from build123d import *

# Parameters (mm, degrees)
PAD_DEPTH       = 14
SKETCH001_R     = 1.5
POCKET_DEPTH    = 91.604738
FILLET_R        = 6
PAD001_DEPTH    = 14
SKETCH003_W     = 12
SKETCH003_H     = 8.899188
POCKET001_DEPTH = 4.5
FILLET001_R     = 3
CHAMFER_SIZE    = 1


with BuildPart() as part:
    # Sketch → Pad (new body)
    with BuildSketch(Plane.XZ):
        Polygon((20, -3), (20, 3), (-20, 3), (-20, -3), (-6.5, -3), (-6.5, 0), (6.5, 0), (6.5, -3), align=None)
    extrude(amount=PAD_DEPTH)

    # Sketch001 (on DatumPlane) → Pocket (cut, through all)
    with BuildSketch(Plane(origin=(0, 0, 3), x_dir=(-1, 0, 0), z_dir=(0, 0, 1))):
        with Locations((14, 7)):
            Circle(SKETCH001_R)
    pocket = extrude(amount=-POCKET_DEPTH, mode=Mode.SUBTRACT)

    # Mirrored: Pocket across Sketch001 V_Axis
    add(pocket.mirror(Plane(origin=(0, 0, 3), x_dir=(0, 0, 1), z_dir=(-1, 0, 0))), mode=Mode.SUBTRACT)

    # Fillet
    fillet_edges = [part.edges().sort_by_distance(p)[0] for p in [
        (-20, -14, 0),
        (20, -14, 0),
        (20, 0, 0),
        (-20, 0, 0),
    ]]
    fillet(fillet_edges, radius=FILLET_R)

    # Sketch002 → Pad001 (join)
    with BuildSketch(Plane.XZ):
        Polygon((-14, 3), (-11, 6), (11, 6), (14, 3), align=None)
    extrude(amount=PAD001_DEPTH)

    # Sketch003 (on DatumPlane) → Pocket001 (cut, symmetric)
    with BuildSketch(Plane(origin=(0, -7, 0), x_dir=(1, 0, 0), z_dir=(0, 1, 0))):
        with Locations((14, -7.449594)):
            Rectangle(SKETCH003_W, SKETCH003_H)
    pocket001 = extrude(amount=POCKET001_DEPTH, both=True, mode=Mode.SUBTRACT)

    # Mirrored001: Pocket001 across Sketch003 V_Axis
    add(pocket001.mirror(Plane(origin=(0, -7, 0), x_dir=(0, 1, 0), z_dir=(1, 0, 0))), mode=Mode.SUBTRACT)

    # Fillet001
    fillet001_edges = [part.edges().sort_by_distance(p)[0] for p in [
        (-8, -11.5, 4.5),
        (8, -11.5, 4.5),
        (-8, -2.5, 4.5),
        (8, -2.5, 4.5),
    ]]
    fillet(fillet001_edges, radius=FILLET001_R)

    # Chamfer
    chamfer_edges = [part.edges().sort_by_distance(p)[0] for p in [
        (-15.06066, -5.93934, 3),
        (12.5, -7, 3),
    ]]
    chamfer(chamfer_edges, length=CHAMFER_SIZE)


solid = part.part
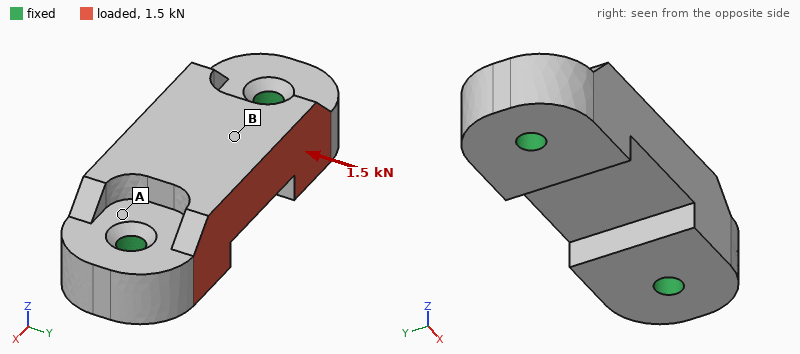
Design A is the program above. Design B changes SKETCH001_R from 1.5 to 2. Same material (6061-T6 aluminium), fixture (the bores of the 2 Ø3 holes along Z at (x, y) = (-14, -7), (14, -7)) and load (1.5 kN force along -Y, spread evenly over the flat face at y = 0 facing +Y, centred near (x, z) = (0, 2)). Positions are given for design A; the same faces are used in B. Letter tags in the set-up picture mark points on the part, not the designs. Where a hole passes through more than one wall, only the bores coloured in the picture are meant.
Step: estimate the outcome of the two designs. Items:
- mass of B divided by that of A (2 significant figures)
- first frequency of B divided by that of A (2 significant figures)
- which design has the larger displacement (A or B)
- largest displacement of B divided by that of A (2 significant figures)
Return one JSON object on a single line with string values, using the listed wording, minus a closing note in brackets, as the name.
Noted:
{"mass of B divided by that of A": "0.98", "first frequency of B divided by that of A": "1.1", "which design has the larger displacement": "A", "largest displacement of B divided by that of A": "0.82"}
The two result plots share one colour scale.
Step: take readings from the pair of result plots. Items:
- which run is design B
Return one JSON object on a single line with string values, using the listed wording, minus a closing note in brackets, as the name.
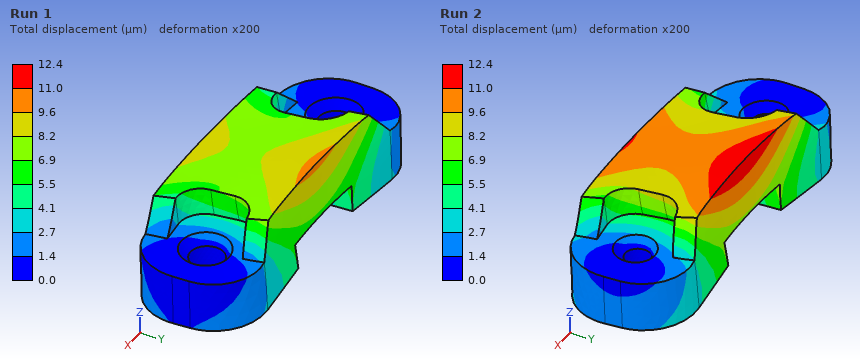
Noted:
{"which run is design B": "Run 1"}
